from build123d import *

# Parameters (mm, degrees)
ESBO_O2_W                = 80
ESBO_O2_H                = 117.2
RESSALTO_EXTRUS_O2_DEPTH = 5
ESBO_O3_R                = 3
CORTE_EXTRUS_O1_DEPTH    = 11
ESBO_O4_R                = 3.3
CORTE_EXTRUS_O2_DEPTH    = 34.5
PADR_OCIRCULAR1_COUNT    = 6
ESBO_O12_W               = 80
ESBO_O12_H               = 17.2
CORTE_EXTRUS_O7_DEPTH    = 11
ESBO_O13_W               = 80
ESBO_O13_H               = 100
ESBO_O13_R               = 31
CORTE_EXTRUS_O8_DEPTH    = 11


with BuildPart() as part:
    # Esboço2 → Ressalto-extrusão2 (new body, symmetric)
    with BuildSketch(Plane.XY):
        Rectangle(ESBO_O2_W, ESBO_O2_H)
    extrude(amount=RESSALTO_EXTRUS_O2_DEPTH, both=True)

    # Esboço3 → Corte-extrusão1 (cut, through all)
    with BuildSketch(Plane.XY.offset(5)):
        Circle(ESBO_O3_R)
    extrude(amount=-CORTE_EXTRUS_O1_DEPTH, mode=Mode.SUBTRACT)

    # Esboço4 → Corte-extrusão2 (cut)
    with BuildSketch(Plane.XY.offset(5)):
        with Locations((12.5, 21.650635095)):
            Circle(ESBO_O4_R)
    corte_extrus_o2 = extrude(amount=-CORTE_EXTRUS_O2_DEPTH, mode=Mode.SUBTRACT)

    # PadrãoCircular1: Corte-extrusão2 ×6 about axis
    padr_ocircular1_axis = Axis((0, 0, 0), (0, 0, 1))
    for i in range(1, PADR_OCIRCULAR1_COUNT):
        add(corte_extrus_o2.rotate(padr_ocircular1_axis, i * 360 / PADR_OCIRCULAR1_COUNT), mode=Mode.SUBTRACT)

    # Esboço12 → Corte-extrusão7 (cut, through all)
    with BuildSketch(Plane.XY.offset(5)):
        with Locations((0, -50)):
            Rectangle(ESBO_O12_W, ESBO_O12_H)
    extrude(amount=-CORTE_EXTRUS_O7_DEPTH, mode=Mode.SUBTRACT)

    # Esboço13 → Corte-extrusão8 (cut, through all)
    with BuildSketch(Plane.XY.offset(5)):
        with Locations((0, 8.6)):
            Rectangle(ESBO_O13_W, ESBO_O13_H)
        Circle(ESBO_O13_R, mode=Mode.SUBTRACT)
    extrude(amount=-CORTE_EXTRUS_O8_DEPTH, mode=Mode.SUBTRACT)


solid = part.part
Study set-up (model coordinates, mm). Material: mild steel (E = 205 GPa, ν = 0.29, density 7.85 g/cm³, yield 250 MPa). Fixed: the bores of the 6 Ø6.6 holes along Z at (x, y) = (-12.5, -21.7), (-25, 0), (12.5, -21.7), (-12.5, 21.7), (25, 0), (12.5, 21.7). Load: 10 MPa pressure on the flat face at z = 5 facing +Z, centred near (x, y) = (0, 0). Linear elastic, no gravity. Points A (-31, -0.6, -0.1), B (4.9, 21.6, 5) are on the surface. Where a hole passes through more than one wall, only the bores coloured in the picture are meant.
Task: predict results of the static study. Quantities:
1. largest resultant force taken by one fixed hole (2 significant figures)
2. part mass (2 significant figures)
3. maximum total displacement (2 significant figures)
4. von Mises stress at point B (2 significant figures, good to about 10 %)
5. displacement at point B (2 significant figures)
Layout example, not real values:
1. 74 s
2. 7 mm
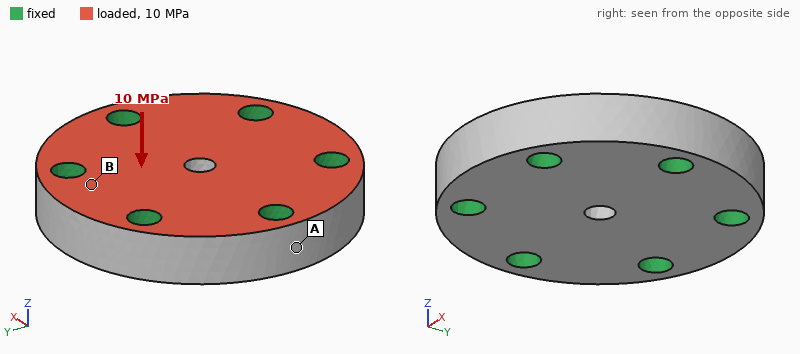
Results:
1. 4.7 kN
2. 220 g
3. 5.6 µm
4. 23 MPa
5. 1.5 µm
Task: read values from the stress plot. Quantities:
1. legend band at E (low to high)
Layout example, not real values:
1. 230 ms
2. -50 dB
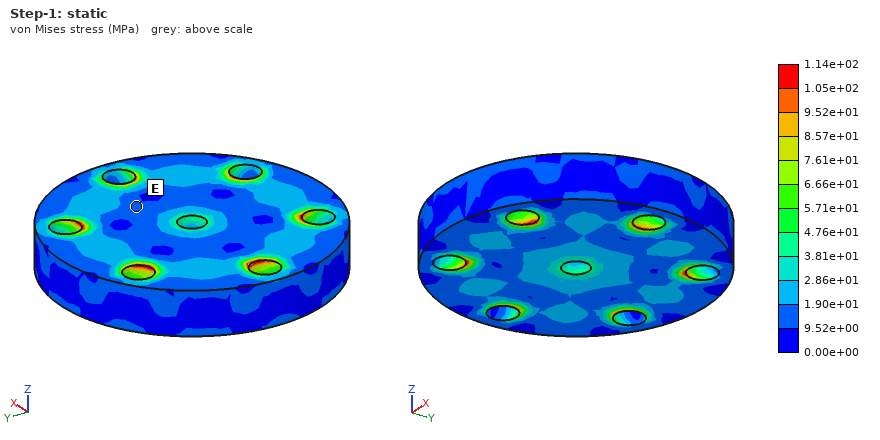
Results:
1. 9.52e+00 to 1.90e+01 MPa
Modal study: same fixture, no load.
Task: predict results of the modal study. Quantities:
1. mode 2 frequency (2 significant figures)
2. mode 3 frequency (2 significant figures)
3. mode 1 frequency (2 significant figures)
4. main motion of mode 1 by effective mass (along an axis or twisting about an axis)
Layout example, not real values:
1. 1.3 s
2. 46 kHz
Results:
1. 49 kHz
2. 49 kHz
3. 29 kHz
4. along Z
